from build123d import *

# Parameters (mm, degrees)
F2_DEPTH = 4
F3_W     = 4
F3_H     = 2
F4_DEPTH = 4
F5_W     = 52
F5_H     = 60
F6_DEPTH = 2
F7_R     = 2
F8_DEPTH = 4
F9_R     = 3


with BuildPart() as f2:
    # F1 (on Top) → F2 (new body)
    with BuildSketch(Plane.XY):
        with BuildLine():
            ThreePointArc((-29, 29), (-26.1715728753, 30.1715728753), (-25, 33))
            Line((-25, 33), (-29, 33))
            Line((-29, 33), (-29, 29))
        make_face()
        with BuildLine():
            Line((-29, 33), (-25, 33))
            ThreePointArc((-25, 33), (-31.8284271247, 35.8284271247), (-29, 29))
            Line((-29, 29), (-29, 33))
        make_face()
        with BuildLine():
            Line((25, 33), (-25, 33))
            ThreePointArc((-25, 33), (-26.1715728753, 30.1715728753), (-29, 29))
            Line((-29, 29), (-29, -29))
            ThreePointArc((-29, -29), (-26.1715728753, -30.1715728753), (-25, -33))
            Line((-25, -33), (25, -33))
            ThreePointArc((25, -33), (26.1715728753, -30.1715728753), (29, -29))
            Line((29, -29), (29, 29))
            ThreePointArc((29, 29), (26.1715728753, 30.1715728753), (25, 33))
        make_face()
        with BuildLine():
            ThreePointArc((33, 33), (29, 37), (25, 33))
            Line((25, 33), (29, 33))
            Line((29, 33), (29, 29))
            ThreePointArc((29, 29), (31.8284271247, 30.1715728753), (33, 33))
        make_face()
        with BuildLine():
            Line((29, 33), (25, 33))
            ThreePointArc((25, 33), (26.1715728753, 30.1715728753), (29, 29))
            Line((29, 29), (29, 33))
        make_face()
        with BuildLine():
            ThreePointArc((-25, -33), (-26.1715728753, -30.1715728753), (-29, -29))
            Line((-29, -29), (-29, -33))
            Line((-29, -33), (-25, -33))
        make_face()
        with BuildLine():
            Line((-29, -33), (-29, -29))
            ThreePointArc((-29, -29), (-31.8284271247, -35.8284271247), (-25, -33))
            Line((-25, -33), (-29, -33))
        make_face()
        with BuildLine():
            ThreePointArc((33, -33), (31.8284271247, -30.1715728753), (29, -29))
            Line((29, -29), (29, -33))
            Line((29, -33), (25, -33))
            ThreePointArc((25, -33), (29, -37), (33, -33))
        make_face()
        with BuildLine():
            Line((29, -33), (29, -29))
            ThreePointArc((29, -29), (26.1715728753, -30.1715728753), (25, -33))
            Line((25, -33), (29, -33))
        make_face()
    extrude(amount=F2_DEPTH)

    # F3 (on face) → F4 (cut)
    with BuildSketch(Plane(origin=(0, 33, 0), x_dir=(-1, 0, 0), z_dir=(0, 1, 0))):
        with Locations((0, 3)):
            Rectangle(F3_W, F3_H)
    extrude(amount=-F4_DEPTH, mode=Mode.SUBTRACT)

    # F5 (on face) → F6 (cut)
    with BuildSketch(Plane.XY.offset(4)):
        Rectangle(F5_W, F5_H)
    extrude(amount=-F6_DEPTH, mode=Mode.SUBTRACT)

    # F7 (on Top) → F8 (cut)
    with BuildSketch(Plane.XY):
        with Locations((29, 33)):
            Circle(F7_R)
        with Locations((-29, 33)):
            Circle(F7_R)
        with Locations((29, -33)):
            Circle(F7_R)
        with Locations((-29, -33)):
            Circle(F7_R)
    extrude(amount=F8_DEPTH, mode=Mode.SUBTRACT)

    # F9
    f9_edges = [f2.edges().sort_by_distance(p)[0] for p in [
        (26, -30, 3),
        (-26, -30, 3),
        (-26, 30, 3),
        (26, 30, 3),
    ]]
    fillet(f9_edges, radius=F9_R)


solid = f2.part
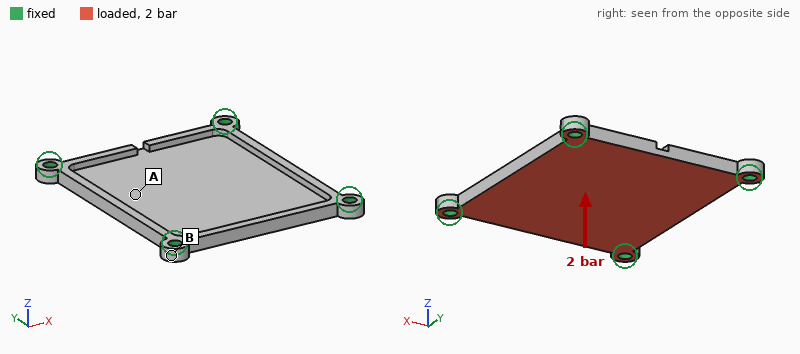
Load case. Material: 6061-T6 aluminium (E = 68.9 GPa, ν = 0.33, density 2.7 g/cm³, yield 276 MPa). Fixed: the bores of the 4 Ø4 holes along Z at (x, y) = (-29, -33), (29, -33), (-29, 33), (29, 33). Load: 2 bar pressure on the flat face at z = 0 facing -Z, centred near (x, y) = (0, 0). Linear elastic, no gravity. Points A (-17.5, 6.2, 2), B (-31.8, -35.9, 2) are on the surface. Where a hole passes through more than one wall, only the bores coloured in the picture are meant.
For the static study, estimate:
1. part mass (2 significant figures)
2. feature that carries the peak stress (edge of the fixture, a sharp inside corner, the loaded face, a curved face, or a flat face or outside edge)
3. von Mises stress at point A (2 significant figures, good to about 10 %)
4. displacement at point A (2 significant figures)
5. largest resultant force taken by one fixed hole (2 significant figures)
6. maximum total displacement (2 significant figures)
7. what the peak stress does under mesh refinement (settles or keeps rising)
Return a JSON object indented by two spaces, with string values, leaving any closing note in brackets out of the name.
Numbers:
{
  "part mass": "26 g",
  "feature that carries the peak stress": "edge of the fixture",
  "von Mises stress at point A": "25 MPa",
  "displacement at point A": "0.15 mm",
  "largest resultant force taken by one fixed hole": "360 N",
  "maximum total displacement": "0.22 mm",
  "what the peak stress does under mesh refinement": "keeps rising"
}
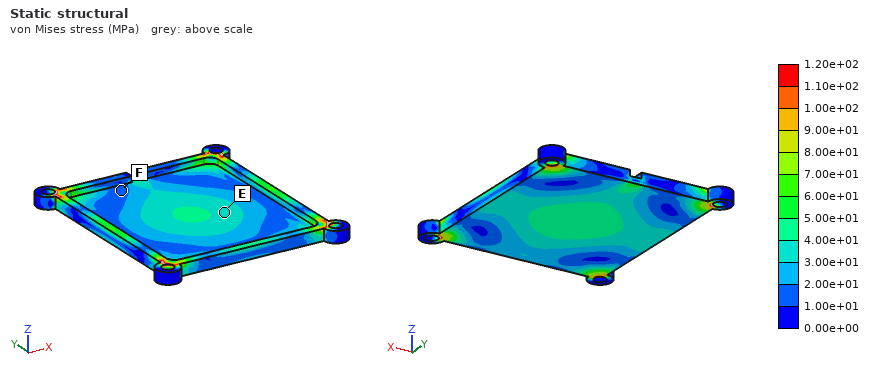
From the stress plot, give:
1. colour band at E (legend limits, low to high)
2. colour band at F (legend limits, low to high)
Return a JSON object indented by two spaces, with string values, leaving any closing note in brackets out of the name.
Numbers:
{
  "colour band at E": "3.00e+01 to 4.00e+01 MPa",
  "colour band at F": "1.00e+01 to 2.00e+01 MPa"
}
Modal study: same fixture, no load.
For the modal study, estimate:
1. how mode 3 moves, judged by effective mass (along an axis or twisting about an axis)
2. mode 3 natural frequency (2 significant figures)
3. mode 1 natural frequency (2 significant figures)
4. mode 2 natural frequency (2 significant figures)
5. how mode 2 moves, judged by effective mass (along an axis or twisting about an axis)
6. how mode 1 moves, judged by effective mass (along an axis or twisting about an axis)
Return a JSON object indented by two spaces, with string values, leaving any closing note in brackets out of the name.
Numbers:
{
  "how mode 3 moves, judged by effective mass": "twisting about X",
  "mode 3 natural frequency": "4800 Hz",
  "mode 1 natural frequency": "2500 Hz",
  "mode 2 natural frequency": "4400 Hz",
  "how mode 2 moves, judged by effective mass": "twisting about Y",
  "how mode 1 moves, judged by effective mass": "along Z"
}
